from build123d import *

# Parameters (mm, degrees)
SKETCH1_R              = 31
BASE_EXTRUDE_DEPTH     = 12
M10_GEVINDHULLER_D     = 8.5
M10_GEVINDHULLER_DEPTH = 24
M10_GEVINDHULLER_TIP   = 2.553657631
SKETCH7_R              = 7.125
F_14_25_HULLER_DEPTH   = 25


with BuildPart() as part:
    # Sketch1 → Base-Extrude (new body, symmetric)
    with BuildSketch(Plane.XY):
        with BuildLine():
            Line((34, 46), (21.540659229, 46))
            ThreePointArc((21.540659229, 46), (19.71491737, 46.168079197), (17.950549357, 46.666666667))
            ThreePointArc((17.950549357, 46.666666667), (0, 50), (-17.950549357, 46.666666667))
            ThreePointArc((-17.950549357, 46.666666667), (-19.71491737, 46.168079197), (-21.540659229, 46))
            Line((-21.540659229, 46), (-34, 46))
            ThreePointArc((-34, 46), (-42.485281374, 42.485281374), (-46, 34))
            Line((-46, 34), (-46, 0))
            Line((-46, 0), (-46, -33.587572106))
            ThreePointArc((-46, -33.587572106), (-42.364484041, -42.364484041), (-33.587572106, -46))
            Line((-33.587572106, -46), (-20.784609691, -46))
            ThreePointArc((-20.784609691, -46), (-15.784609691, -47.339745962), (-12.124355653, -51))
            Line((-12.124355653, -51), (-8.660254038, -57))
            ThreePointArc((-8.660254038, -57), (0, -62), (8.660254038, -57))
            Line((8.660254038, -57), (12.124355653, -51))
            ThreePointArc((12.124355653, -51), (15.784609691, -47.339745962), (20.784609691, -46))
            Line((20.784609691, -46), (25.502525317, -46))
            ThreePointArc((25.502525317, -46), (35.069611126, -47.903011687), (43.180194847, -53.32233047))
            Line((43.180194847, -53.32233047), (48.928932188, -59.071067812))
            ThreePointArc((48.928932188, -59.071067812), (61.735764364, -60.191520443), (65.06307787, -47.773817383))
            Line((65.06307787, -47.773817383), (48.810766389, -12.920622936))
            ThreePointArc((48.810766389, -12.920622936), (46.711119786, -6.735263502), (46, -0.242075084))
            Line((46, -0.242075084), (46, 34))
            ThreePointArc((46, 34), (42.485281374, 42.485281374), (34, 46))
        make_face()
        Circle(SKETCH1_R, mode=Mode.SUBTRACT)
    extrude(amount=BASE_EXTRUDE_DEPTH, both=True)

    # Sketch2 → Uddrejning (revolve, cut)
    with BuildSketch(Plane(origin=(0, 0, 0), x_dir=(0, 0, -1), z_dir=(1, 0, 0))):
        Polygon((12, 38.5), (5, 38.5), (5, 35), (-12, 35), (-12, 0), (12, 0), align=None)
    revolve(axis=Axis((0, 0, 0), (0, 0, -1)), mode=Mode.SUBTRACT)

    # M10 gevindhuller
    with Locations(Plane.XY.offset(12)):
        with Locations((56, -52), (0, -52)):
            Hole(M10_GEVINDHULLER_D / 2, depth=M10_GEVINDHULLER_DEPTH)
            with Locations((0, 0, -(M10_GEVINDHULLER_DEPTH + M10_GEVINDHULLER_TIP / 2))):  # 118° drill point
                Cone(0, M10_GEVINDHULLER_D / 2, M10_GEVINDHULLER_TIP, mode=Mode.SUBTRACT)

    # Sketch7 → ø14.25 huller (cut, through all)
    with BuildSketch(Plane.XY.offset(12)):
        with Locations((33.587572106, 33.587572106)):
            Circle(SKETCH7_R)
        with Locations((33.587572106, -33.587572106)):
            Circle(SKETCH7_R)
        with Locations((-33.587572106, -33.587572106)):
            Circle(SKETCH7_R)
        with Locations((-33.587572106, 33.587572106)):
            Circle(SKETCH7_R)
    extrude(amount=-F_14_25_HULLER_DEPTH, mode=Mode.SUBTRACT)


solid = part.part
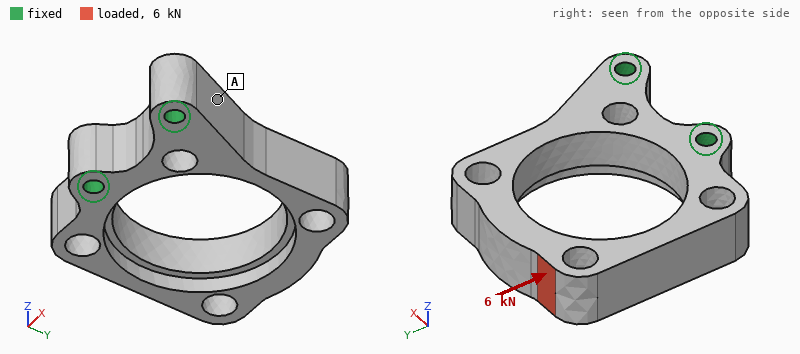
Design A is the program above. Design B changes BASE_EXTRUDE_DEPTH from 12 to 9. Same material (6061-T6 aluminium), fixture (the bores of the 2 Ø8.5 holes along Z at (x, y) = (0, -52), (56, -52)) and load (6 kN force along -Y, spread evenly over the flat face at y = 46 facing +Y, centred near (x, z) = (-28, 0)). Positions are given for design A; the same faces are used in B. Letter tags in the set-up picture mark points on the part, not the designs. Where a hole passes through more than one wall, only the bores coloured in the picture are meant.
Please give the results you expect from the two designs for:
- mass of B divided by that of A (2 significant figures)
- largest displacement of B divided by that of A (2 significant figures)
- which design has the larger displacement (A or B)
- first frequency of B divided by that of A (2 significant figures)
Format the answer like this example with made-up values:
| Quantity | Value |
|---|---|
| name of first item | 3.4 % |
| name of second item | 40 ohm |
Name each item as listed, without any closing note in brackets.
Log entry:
| Quantity | Value |
|---|---|
| mass of B divided by that of A | 0.76 |
| largest displacement of B divided by that of A | 1.3 |
| which design has the larger displacement | B |
| first frequency of B divided by that of A | 0.80 |
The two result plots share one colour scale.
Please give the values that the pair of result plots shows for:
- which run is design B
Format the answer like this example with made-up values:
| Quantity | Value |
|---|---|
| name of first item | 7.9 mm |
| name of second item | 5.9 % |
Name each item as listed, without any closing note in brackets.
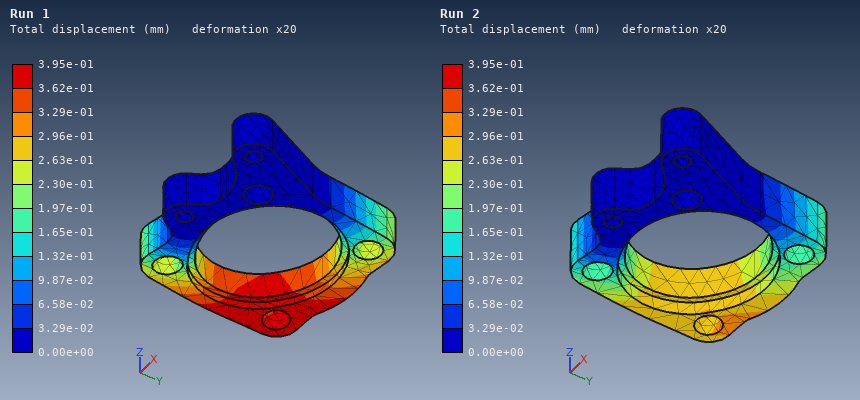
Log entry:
| Quantity | Value |
|---|---|
| which run is design B | Run 1 |
